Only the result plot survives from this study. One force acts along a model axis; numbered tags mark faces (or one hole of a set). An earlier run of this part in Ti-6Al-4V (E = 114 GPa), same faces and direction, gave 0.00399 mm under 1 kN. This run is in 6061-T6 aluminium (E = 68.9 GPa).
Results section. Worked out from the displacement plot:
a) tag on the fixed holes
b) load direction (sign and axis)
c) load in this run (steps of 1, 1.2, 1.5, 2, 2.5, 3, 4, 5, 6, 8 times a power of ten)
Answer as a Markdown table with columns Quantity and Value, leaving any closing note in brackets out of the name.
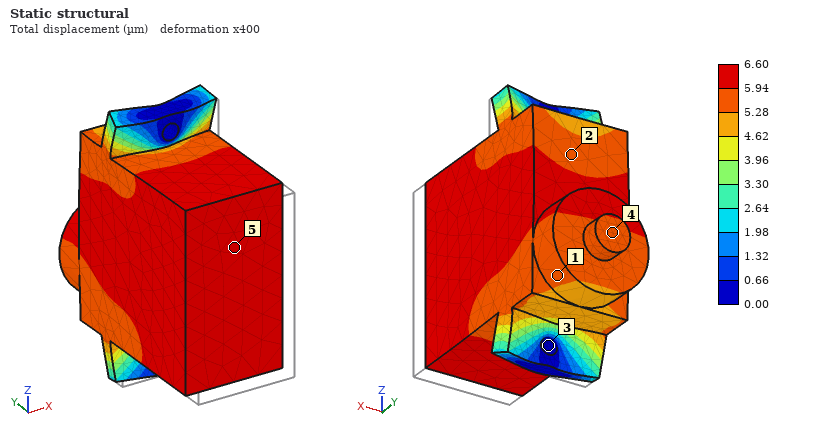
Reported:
| Quantity | Value |
|---|---|
| tag on the fixed holes | 3 |
| load direction | +Y |
| load in this run | 1 kN |
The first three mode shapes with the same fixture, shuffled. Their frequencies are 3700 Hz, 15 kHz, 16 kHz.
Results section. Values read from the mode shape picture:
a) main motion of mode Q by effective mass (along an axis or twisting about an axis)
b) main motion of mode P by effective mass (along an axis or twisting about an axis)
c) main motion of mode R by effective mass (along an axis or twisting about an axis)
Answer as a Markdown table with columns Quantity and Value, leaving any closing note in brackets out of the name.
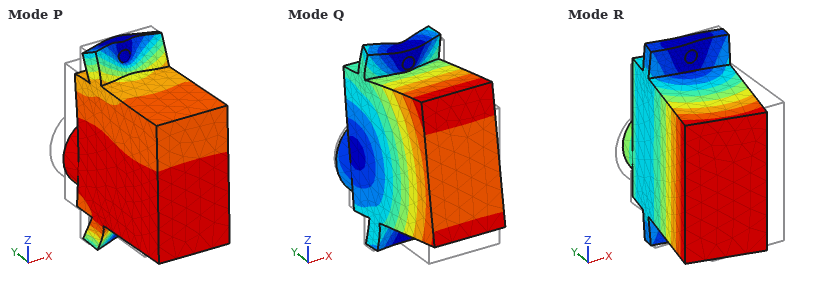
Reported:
| Quantity | Value |
|---|---|
| main motion of mode Q by effective mass | along Z |
| main motion of mode P by effective mass | along Y |
| main motion of mode R by effective mass | along X |
